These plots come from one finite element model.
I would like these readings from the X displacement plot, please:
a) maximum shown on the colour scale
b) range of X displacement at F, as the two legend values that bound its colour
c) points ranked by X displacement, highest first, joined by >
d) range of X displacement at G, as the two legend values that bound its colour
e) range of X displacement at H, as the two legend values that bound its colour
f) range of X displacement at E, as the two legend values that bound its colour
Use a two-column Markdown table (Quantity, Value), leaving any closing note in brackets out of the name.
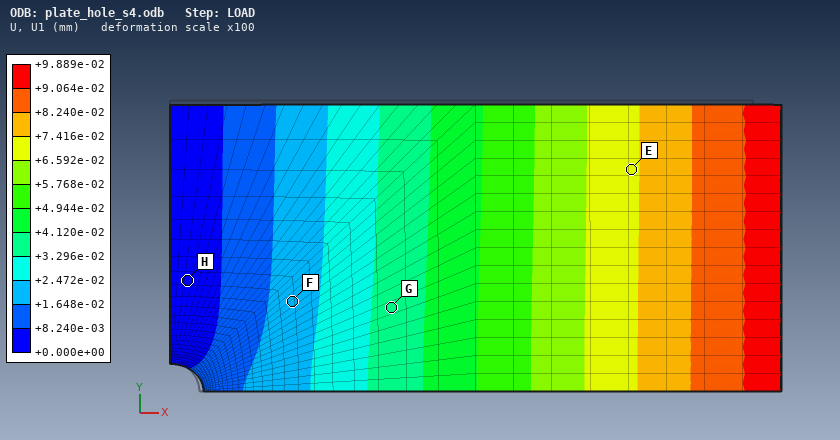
| Quantity | Value |
|---|---|
| maximum shown on the colour scale | +9.889e-02 mm |
| range of X displacement at F, as the two legend values that bound its colour | +1.648e-02 to +2.472e-02 mm |
| points ranked by X displacement, highest first, joined by > | E > G > F > H |
| range of X displacement at G, as the two legend values that bound its colour | +3.296e-02 to +4.120e-02 mm |
| range of X displacement at H, as the two legend values that bound its colour | +0.000e+00 to +8.240e-03 mm |
| range of X displacement at E, as the two legend values that bound its colour | +6.592e-02 to +7.416e-02 mm |
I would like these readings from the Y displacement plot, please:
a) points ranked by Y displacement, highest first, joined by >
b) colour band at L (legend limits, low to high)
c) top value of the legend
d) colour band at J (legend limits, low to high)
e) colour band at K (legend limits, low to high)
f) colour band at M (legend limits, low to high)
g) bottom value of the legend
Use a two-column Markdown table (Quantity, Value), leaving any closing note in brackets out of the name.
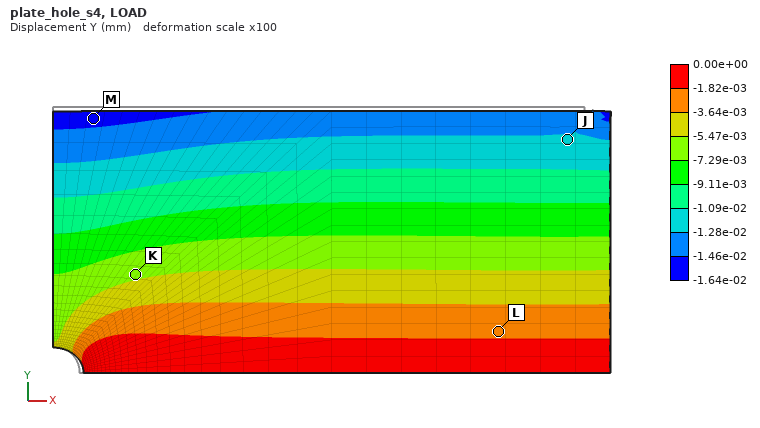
| Quantity | Value |
|---|---|
| points ranked by Y displacement, highest first, joined by > | L > K > J > M |
| colour band at L | -3.64e-03 to -1.82e-03 mm |
| top value of the legend | 0.00e+00 mm |
| colour band at J | -1.28e-02 to -1.09e-02 mm |
| colour band at K | -7.29e-03 to -5.47e-03 mm |
| colour band at M | -1.64e-02 to -1.46e-02 mm |
| bottom value of the legend | -1.64e-02 mm |
